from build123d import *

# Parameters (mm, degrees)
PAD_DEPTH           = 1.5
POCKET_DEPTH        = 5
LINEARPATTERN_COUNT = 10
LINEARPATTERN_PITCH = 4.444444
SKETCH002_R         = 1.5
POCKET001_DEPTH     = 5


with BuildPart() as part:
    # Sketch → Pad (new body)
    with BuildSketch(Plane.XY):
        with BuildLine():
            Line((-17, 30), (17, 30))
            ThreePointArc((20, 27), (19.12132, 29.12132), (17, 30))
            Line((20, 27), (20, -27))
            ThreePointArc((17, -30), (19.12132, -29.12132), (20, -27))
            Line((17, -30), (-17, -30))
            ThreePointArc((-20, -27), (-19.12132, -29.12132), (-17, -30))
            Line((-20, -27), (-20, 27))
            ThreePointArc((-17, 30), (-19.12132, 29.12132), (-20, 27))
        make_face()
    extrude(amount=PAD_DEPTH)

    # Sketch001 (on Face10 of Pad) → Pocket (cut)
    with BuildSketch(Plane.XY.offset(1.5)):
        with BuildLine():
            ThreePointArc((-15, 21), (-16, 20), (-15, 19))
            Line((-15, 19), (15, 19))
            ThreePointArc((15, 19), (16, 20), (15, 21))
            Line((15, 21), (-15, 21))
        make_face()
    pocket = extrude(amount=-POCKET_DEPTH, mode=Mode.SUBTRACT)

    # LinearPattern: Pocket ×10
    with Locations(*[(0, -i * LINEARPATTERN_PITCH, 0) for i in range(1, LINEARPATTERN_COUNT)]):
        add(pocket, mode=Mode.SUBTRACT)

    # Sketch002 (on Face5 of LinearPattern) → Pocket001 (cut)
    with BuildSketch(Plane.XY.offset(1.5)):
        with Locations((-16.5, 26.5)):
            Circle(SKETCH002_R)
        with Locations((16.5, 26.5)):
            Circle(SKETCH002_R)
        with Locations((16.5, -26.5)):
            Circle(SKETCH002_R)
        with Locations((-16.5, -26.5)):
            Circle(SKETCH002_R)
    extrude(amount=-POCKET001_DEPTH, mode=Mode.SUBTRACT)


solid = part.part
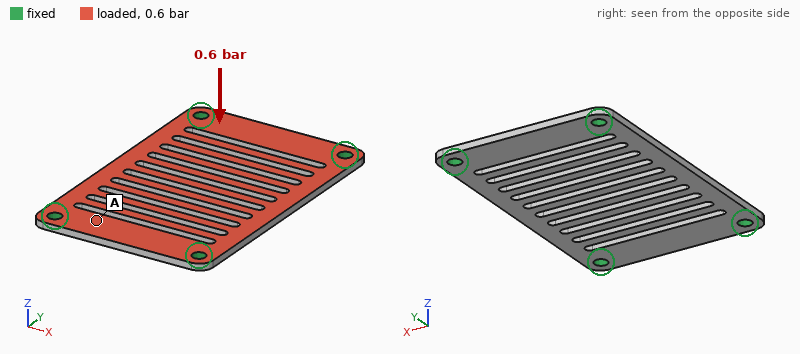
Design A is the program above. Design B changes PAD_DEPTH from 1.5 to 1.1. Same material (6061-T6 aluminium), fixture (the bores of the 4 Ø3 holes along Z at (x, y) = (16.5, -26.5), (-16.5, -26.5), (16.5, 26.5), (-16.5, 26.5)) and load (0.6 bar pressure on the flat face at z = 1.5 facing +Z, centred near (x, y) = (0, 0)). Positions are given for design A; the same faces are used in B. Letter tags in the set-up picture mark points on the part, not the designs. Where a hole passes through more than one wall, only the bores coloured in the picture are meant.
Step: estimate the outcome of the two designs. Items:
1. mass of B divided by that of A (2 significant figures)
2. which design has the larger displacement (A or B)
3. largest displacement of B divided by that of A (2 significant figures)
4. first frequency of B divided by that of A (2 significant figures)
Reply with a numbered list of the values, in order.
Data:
1. 0.73
2. B
3. 2.5
4. 0.74
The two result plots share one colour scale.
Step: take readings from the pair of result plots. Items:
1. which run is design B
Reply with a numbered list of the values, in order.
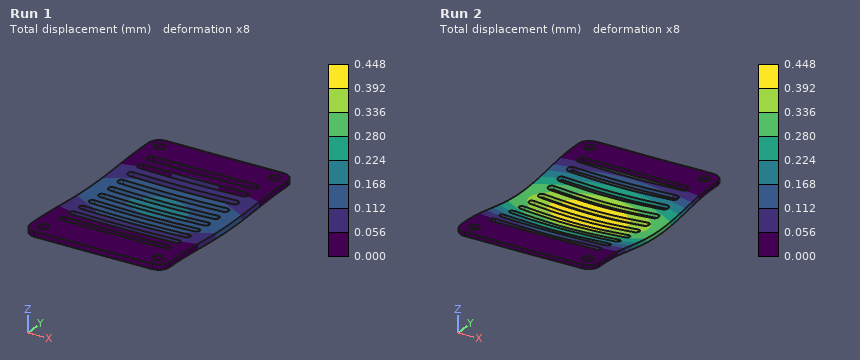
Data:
1. Run 2
